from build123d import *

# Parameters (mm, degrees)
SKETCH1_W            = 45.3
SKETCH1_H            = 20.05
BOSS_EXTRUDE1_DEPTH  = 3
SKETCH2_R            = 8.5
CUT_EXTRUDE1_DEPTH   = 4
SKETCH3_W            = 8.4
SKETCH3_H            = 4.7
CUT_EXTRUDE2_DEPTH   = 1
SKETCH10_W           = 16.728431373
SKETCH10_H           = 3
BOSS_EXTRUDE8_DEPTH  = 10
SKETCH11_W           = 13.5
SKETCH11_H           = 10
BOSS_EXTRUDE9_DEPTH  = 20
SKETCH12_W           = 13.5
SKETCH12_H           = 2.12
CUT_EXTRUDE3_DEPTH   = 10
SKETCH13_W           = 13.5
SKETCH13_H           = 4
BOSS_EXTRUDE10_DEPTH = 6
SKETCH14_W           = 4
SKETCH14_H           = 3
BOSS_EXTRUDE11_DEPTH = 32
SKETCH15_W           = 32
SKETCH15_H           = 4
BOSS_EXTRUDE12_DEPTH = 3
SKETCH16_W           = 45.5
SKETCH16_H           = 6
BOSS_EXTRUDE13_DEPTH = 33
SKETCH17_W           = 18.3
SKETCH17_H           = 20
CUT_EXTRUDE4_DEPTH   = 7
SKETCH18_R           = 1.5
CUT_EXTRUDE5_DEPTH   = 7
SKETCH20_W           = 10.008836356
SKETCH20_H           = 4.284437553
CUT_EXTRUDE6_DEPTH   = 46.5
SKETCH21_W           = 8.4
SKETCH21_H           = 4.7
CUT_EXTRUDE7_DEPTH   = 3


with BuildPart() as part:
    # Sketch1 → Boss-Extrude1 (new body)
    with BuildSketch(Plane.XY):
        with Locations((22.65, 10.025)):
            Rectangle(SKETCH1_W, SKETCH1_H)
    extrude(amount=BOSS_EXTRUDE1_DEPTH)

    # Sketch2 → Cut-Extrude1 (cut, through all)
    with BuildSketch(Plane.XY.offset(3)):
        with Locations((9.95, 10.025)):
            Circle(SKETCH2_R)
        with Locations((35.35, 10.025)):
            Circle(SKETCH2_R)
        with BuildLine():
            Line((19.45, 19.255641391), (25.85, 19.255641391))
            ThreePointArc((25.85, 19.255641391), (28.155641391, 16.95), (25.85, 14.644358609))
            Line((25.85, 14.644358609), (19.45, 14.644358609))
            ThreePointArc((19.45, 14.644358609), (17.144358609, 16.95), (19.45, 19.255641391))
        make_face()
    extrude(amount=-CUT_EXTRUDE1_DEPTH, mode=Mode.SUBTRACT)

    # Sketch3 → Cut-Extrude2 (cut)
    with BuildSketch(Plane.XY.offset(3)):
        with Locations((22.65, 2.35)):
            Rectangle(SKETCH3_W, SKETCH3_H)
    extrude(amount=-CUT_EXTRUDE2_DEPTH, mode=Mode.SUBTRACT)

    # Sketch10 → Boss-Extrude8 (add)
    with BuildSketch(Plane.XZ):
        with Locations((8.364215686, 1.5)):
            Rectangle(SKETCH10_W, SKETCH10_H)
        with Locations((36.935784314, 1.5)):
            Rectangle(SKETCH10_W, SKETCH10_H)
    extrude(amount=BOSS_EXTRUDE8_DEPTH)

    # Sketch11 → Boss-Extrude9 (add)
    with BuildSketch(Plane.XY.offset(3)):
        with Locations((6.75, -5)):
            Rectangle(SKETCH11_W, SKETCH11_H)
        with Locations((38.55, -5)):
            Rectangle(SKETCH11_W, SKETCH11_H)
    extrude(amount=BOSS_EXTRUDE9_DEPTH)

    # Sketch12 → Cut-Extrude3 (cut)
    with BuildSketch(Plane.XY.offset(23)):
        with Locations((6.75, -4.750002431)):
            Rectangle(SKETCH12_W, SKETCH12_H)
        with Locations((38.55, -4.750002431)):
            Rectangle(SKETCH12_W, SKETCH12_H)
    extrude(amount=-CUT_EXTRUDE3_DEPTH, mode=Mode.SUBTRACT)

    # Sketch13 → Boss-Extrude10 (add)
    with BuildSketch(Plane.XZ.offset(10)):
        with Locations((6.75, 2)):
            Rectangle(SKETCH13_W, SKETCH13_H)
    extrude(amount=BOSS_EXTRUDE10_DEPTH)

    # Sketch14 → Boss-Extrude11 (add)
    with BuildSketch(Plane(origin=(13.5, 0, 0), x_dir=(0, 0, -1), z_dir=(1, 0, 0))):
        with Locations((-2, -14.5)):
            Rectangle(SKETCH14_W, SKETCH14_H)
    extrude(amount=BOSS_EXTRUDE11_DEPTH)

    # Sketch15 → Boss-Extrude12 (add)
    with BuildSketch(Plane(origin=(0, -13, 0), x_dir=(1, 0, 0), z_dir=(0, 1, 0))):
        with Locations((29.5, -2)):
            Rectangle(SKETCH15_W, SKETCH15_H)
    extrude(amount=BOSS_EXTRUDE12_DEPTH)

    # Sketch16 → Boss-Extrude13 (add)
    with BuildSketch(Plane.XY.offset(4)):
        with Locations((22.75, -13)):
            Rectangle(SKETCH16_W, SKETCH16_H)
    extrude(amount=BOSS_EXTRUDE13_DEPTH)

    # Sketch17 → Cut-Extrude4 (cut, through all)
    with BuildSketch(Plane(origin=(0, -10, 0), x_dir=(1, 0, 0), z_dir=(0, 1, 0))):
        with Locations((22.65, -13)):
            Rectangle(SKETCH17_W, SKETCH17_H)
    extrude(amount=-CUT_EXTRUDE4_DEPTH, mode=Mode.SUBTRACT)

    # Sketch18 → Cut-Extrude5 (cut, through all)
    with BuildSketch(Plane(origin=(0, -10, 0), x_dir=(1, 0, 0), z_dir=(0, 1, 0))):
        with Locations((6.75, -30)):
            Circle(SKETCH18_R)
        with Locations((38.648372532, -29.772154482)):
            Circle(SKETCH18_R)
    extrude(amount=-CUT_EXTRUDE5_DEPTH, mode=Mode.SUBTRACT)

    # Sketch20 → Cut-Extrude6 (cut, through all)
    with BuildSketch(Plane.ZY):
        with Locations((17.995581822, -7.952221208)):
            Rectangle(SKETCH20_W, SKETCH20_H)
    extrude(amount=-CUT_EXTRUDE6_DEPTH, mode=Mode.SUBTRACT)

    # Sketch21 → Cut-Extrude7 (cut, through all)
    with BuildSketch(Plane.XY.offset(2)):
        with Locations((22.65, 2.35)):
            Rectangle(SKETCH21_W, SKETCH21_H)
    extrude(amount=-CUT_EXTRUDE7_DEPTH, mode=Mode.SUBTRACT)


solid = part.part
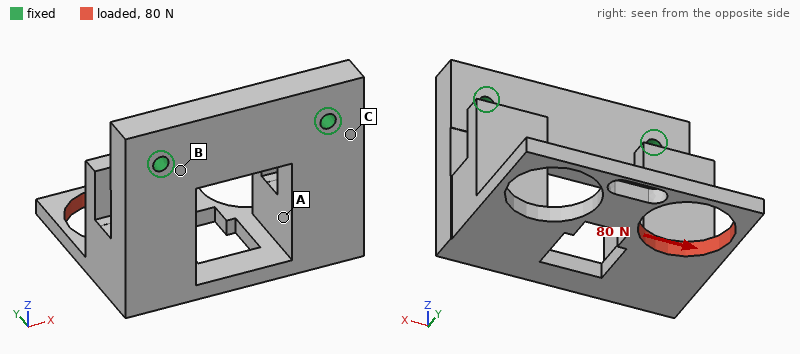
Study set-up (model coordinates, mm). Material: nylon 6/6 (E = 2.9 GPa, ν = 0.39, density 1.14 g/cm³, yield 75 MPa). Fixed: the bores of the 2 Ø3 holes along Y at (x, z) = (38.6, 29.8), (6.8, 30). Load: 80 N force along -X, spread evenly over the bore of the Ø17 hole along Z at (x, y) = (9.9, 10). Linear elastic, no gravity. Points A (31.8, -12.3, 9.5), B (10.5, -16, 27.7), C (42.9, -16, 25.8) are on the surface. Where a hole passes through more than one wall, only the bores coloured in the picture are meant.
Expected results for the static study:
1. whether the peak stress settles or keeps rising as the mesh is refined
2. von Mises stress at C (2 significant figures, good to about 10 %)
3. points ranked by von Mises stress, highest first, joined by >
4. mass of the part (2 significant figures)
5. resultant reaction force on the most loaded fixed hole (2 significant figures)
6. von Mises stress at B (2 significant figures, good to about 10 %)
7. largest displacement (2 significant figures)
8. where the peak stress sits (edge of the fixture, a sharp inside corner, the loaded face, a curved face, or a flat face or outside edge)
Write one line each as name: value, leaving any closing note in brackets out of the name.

whether the peak stress settles or keeps rising as the mesh is refined: keeps rising
von Mises stress at C: 8.3 MPa
points ranked by von Mises stress, highest first, joined by >: C > B > A
mass of the part: 16 g
resultant reaction force on the most loaded fixed hole: 84 N
von Mises stress at B: 4.0 MPa
largest displacement: 0.68 mm
where the peak stress sits: edge of the fixture
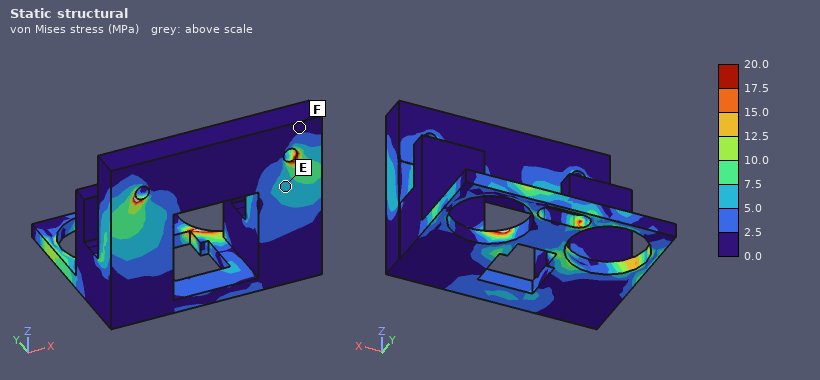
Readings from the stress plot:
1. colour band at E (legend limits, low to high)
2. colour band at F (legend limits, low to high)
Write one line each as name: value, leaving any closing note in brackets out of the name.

colour band at E: 5.0 to 7.5 MPa
colour band at F: 0.0 to 2.5 MPa
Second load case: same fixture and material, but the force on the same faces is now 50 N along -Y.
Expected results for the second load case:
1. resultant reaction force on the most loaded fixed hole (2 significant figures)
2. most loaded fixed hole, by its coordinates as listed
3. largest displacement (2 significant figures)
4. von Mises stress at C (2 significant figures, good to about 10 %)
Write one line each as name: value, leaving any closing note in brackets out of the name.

resultant reaction force on the most loaded fixed hole: 40 N
most loaded fixed hole, by its coordinates as listed: (6.8, 30)
largest displacement: 0.71 mm
von Mises stress at C: 4.1 MPa
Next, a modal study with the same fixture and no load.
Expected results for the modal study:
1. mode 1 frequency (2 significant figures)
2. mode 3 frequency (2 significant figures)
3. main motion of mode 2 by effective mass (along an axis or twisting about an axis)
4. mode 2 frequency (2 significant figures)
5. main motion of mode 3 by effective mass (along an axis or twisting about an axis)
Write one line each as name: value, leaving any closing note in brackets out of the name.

mode 1 frequency: 700 Hz
mode 3 frequency: 1300 Hz
main motion of mode 2 by effective mass: along X
mode 2 frequency: 1100 Hz
main motion of mode 3 by effective mass: along Y
